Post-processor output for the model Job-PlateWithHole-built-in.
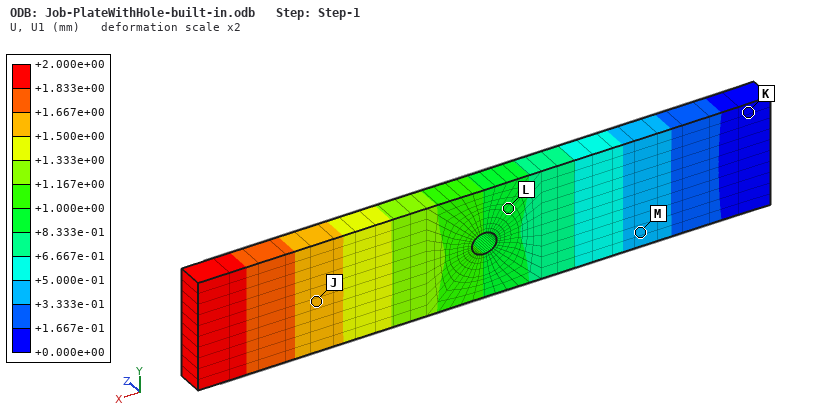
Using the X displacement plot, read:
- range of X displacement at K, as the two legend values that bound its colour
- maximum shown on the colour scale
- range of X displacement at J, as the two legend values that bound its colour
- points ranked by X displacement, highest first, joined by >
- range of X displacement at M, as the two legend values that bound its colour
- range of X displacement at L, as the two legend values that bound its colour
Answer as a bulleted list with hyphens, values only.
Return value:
- +0.000e+00 to +1.667e-01 mm
- +2.000e+00 mm
- +1.500e+00 to +1.667e+00 mm
- J > L > M > K
- +3.333e-01 to +5.000e-01 mm
- +8.333e-01 to +1.000e+00 mm
